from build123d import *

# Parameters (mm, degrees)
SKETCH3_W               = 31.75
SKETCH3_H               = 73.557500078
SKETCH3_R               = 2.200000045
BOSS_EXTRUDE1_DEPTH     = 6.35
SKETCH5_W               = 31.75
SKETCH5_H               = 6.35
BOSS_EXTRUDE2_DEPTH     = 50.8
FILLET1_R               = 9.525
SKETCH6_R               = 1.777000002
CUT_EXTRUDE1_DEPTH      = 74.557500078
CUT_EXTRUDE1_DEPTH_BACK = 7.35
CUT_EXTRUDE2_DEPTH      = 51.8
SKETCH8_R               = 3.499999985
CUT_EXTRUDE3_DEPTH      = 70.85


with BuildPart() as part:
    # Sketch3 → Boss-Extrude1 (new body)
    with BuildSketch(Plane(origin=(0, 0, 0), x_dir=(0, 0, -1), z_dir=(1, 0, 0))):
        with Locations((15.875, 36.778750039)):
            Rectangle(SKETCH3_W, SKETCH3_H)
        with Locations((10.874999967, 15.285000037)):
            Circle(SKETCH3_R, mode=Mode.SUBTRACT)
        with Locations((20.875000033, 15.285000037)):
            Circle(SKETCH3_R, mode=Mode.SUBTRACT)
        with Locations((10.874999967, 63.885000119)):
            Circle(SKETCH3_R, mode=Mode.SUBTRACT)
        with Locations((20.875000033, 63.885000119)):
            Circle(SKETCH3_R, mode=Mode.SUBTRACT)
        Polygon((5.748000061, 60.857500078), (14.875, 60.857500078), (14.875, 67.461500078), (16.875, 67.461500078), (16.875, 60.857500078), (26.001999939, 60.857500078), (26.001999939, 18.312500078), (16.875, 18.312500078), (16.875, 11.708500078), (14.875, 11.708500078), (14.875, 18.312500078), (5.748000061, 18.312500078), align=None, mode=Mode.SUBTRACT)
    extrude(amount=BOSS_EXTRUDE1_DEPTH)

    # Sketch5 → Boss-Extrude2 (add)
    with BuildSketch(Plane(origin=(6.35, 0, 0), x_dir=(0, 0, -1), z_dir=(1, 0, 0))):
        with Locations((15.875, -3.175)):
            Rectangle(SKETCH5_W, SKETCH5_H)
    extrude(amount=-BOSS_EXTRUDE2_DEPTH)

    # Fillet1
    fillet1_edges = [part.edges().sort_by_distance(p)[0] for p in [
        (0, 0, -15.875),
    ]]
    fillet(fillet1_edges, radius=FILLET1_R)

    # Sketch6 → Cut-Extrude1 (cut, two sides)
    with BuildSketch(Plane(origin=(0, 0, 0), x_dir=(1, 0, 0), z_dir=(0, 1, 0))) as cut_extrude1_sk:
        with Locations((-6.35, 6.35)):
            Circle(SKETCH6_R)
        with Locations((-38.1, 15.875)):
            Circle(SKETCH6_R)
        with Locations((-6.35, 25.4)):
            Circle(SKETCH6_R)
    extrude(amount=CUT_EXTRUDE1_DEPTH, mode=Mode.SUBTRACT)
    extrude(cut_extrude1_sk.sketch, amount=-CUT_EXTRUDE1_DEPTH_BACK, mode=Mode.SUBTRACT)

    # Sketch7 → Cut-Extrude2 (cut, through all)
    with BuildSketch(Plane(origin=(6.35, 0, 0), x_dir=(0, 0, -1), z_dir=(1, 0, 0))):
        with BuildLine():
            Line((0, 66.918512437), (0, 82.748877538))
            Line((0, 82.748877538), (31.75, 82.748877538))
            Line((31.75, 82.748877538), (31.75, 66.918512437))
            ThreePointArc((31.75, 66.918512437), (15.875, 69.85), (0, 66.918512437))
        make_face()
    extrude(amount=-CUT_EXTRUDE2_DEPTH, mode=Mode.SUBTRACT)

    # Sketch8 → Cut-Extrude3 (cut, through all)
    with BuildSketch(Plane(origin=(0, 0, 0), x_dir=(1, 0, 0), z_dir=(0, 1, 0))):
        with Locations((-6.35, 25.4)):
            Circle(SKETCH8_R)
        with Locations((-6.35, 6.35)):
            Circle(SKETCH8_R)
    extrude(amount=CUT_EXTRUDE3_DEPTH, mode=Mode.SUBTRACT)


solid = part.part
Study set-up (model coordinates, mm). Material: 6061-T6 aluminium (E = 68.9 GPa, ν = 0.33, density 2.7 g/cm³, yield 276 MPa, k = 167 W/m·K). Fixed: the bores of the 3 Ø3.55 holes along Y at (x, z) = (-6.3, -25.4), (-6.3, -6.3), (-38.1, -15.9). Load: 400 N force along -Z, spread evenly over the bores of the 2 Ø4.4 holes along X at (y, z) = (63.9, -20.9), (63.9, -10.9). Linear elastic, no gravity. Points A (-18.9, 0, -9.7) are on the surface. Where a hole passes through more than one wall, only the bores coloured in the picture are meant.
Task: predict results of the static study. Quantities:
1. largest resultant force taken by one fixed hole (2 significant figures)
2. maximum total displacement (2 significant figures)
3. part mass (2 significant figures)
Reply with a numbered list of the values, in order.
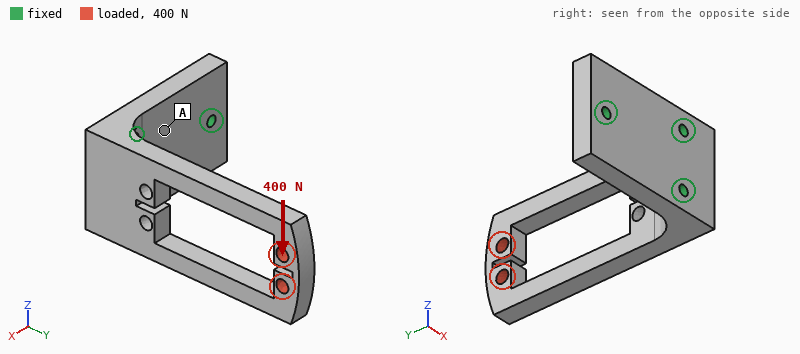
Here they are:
1. 1.2 kN
2. 0.45 mm
3. 50 g
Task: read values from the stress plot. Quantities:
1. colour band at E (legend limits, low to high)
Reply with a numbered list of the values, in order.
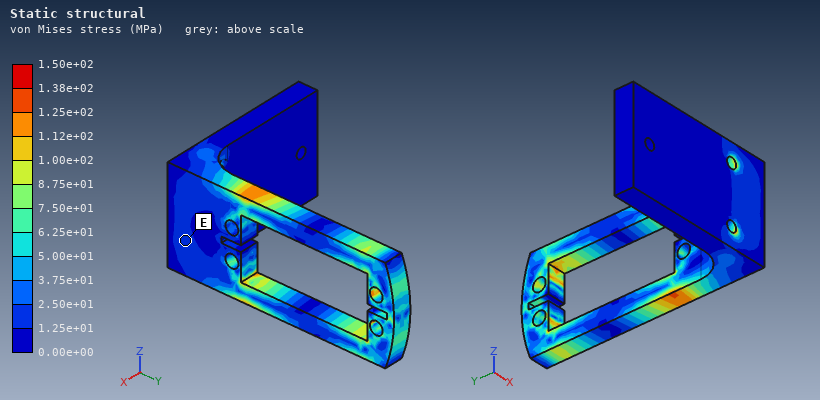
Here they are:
1. 1.25e+01 to 2.50e+01 MPa
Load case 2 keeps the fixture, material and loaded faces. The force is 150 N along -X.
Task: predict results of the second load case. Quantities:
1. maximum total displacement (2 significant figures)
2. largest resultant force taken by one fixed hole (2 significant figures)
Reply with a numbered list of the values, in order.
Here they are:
1. 0.66 mm
2. 86 N
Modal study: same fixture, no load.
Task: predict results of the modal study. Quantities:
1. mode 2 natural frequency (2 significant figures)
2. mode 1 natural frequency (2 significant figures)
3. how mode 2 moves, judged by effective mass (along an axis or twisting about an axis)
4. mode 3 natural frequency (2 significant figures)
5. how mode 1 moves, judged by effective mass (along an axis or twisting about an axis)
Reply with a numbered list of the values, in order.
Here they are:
1. 1900 Hz
2. 1000 Hz
3. along Z
4. 3000 Hz
5. along X
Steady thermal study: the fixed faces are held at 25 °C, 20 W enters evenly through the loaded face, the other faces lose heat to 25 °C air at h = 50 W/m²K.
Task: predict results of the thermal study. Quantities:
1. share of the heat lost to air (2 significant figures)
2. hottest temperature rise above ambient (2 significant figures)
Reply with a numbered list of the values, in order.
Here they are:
1. 38 %
2. 77 K
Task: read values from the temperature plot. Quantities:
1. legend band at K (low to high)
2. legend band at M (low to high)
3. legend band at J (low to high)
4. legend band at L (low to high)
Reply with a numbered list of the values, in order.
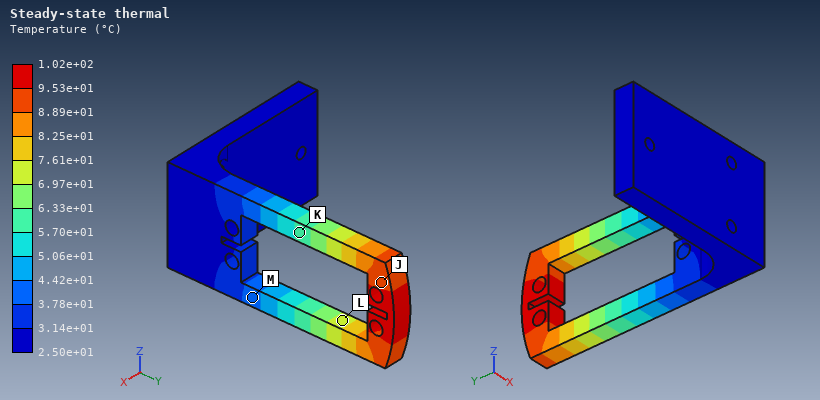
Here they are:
1. 5.70e+01 to 6.33e+01 °C
2. 3.78e+01 to 4.42e+01 °C
3. 8.89e+01 to 9.53e+01 °C
4. 6.97e+01 to 7.61e+01 °C
